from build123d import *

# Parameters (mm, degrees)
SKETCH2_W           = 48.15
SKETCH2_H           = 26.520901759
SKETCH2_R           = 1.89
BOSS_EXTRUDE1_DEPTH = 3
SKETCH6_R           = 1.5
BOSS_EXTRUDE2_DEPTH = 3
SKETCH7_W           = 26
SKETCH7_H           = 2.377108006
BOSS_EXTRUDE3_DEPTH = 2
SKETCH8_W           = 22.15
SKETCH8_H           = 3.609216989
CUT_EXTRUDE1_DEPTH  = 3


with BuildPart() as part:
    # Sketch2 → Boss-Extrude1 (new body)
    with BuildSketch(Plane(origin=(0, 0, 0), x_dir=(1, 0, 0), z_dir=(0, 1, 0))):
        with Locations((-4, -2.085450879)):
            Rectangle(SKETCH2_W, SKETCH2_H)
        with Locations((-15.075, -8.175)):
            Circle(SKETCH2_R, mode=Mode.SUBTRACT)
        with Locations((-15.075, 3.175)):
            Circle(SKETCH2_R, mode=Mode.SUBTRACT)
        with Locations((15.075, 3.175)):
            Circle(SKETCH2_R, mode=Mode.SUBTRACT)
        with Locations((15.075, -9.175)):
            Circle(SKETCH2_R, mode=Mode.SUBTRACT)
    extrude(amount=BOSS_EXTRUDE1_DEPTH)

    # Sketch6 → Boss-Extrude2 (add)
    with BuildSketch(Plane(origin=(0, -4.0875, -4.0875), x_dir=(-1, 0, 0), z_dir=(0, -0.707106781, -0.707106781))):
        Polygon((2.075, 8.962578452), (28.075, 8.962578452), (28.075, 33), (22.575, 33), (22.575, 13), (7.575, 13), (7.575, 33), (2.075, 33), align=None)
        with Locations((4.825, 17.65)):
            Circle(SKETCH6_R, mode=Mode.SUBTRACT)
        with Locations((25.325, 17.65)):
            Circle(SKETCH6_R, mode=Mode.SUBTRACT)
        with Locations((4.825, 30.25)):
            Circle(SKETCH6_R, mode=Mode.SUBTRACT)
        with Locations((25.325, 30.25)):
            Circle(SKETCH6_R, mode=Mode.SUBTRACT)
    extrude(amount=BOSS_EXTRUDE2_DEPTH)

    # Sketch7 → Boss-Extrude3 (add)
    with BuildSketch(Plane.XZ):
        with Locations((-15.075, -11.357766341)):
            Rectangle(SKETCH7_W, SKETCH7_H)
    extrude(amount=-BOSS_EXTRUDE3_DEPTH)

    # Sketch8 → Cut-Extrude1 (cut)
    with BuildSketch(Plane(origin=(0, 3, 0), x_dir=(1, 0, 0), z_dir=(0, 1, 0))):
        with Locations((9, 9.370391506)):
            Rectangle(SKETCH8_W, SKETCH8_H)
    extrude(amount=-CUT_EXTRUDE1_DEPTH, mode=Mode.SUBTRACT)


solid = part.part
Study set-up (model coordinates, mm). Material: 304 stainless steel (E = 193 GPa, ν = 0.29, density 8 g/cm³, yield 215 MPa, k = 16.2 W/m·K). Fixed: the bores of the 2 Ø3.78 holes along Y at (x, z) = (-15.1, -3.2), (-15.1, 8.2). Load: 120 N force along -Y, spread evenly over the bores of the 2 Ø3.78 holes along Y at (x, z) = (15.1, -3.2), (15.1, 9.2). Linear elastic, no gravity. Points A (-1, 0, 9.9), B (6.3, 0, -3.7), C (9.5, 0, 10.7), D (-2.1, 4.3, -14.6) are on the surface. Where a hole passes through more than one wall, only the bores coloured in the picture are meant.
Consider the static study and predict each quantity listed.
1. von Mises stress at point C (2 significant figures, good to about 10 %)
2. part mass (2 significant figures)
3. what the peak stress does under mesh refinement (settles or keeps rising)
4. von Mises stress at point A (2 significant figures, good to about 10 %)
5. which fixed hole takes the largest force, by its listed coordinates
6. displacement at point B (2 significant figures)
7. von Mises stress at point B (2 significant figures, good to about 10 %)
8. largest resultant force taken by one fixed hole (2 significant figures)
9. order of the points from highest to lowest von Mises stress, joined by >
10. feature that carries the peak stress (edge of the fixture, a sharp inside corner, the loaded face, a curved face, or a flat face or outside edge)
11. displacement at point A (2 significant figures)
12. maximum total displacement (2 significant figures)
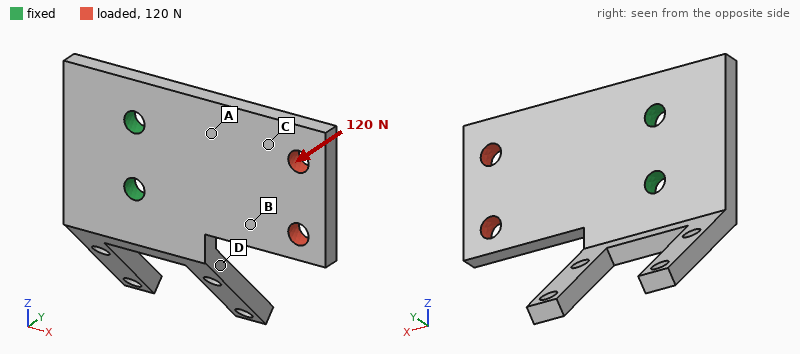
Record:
20 MPa
35 g
keeps rising
49 MPa
(-15.1, 8.2)
0.047 mm
33 MPa
70 N
A > B > C > D
edge of the fixture
0.023 mm
0.11 mm
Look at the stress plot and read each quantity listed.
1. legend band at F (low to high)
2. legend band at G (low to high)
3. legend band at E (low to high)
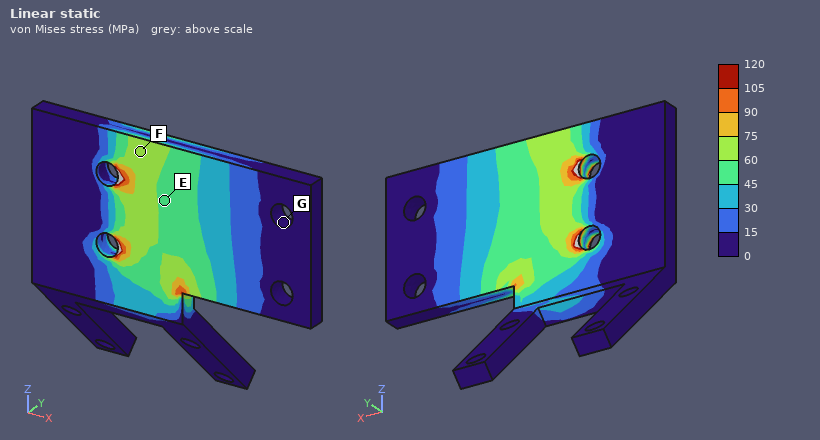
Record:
60 to 75 MPa
0 to 15 MPa
45 to 60 MPa
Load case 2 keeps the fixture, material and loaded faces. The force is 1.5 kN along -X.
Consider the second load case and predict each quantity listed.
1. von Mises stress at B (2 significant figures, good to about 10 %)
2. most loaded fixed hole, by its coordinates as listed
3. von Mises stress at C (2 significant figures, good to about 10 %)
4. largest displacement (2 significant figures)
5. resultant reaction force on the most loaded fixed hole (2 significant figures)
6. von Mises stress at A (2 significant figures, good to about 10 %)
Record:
25 MPa
(-15.1, 8.2)
22 MPa
4.4 µm
810 N
20 MPa
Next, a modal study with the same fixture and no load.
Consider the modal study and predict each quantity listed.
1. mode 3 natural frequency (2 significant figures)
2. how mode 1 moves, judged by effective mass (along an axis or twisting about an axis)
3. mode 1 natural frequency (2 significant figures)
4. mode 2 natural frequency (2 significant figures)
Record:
3300 Hz
along Y
2200 Hz
3200 Hz
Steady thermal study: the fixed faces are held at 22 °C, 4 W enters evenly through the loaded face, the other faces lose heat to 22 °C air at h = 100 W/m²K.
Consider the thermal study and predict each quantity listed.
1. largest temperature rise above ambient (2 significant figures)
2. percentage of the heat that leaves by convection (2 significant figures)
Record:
43 K
82 %
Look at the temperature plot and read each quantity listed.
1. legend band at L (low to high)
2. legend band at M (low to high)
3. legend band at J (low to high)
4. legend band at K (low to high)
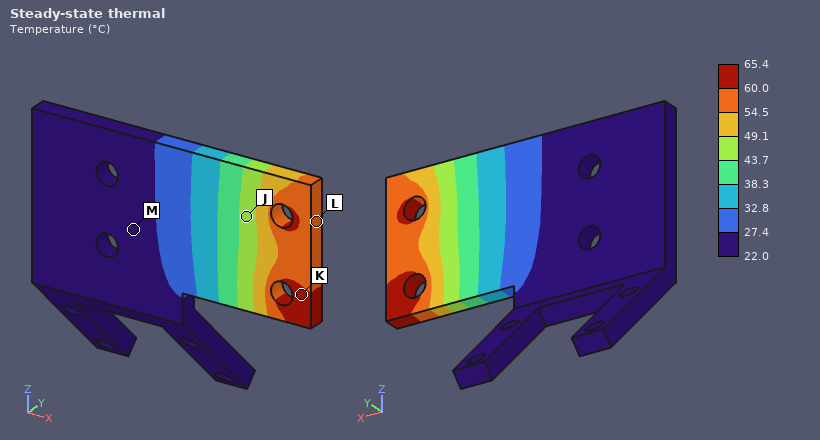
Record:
54.5 to 60.0 °C
22.0 to 27.4 °C
43.7 to 49.1 °C
60.0 to 65.4 °C
